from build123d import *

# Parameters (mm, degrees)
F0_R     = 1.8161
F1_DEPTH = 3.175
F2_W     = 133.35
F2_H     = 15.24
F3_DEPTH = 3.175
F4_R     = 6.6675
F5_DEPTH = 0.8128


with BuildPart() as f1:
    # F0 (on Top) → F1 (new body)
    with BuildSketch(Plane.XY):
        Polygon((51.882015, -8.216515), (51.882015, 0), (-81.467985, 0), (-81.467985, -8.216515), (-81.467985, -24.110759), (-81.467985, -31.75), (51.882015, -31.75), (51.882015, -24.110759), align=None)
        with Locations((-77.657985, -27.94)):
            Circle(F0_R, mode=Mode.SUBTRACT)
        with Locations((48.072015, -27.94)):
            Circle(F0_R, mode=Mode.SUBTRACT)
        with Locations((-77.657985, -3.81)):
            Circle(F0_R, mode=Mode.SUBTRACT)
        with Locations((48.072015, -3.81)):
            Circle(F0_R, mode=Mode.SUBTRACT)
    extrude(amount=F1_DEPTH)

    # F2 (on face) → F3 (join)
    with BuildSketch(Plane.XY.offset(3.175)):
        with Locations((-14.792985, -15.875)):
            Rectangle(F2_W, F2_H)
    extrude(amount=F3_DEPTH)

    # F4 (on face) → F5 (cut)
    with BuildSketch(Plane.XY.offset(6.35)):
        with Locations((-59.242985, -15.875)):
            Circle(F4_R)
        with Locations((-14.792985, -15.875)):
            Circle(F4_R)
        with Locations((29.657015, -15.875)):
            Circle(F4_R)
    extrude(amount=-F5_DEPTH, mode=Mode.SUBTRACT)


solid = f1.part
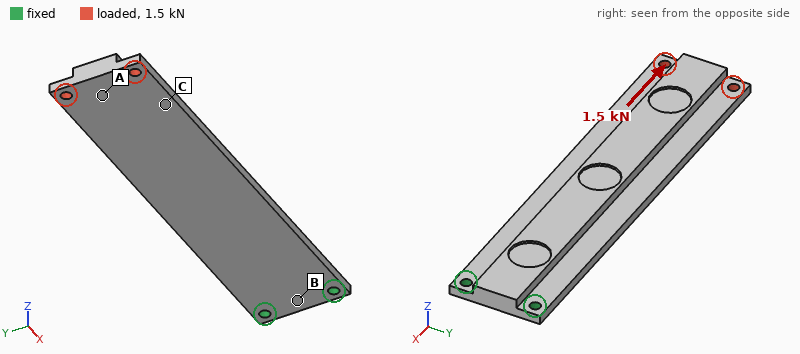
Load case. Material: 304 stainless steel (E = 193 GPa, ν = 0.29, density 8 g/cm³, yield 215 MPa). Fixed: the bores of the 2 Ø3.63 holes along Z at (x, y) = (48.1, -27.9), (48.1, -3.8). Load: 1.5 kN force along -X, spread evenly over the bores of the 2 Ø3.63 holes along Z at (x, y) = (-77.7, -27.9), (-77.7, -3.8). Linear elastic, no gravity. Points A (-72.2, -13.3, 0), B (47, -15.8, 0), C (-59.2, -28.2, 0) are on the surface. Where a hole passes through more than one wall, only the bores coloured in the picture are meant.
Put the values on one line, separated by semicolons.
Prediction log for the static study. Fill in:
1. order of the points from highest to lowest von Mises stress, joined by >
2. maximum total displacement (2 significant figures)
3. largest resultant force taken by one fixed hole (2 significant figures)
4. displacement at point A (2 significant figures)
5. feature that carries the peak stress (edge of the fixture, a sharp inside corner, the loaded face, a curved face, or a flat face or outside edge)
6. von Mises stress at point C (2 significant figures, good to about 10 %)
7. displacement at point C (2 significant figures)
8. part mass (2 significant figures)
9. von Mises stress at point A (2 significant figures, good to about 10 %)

C > A > B; 0.13 mm; 770 N; 0.11 mm; the loaded face; 20 MPa; 0.090 mm; 160 g; 8.6 MPa
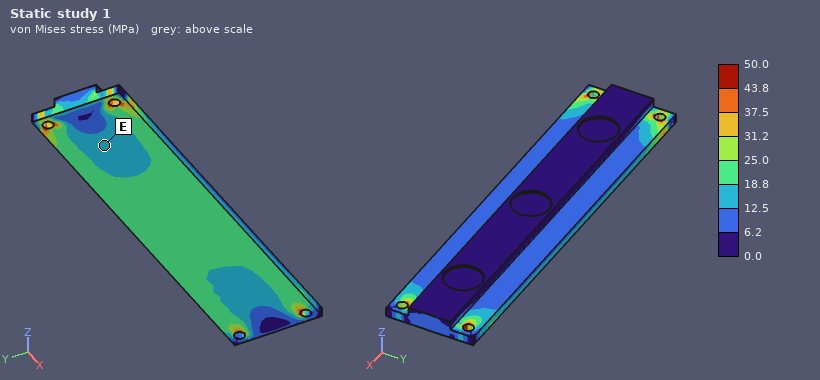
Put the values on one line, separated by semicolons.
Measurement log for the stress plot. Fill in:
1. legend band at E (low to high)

12.5 to 18.8 MPa
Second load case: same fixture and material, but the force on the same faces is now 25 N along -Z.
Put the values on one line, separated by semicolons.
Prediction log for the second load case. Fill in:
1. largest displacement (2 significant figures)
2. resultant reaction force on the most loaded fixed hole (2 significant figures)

0.30 mm; 28 N
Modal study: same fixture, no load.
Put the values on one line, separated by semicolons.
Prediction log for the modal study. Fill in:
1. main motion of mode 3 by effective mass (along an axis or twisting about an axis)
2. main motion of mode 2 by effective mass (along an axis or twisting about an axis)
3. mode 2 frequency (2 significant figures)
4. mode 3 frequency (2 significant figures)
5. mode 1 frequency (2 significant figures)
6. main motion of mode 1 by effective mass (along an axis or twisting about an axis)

along Z; along Y; 1300 Hz; 1500 Hz; 230 Hz; along Z
